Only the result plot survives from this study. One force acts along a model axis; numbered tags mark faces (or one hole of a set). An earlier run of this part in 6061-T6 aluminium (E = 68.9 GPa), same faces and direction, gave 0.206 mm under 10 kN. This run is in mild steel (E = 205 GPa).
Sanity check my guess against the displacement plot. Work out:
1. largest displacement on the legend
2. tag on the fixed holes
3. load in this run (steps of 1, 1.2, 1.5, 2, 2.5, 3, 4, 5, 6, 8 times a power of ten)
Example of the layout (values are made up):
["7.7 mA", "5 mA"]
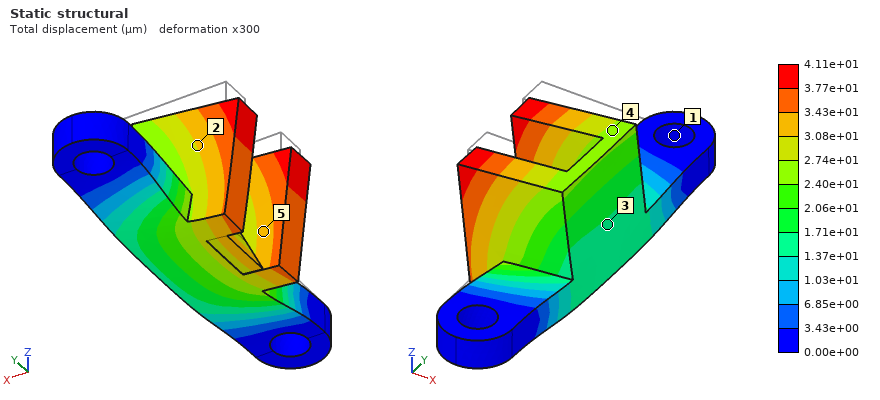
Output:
["4.11e+01 µm", "1", "6 kN"]
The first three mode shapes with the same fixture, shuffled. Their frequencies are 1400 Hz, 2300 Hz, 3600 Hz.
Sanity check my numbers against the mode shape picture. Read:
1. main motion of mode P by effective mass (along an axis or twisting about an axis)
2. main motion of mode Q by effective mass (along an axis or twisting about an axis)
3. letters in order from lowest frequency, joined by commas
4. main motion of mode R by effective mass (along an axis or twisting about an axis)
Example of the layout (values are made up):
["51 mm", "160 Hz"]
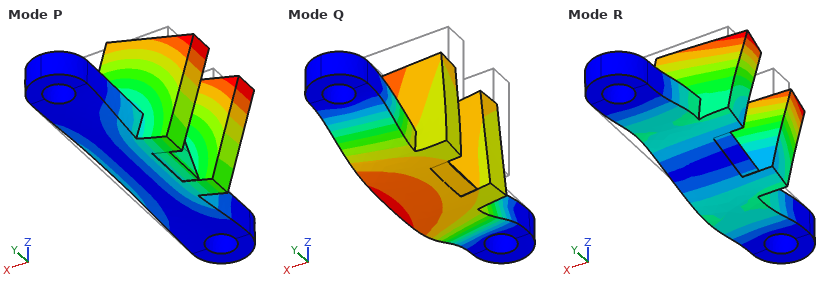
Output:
["along X", "along Z", "P, Q, R", "along Y"]
